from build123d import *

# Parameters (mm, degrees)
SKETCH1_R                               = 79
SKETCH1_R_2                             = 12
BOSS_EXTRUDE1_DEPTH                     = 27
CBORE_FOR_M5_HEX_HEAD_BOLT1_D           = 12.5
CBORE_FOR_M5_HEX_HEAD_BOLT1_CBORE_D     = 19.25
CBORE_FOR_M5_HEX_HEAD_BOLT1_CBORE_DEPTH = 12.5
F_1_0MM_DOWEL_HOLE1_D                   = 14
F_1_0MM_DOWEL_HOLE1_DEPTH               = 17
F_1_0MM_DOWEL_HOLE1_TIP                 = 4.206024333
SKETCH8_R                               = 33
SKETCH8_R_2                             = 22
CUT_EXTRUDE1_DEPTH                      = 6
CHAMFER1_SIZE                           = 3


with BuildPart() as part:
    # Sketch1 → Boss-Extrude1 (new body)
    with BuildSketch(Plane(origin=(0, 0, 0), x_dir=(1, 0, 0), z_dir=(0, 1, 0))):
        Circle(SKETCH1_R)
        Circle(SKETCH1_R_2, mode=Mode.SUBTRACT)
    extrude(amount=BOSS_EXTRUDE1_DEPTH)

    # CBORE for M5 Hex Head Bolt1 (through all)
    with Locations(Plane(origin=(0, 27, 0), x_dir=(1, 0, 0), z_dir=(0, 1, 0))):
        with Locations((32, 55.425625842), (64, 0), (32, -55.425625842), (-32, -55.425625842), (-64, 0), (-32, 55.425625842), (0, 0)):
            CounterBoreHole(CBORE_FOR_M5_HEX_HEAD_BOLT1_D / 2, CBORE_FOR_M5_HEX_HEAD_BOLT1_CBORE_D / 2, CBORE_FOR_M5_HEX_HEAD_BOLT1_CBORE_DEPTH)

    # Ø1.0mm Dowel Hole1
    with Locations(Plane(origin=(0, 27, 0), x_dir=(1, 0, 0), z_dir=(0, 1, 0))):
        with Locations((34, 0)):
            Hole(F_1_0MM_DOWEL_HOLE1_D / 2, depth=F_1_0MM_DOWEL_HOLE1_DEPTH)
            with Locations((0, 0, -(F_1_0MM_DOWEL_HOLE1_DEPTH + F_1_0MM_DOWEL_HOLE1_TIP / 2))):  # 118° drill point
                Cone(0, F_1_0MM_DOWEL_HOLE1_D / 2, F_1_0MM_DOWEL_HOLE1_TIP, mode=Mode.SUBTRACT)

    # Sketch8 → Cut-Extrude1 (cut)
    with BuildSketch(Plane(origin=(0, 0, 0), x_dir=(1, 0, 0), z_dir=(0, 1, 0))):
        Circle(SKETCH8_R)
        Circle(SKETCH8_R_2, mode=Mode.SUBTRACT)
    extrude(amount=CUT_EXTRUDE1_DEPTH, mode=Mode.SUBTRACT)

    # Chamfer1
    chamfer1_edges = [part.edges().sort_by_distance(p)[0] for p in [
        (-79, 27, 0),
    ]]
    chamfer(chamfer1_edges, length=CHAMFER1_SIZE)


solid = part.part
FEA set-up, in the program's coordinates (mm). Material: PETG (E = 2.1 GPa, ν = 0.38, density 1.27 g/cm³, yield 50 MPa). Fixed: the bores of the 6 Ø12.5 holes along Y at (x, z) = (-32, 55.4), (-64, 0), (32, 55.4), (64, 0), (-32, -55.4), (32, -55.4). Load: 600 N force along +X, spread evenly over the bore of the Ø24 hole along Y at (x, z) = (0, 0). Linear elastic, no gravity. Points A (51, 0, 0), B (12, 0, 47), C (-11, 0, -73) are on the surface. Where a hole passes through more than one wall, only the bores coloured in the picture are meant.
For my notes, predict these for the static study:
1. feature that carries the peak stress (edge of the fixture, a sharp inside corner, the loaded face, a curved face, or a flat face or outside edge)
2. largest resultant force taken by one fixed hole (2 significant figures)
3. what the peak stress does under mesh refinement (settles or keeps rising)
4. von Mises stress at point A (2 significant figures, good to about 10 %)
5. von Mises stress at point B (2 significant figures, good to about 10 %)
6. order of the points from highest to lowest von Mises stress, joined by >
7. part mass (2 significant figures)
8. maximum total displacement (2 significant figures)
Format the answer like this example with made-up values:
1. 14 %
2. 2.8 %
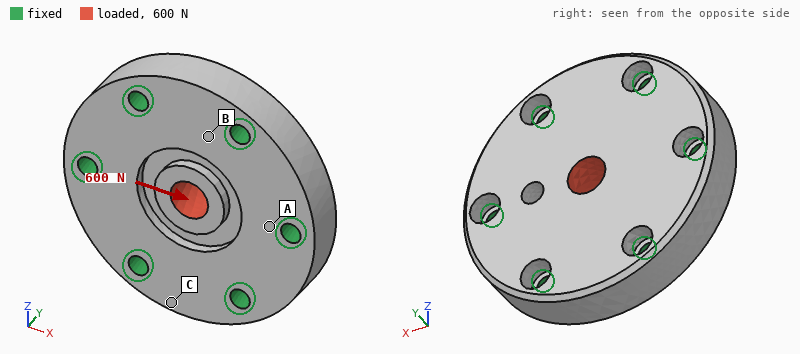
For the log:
1. a sharp inside corner
2. 150 N
3. keeps rising
4. 0.23 MPa
5. 0.12 MPa
6. A > B > C
7. 590 g
8. 10 µm
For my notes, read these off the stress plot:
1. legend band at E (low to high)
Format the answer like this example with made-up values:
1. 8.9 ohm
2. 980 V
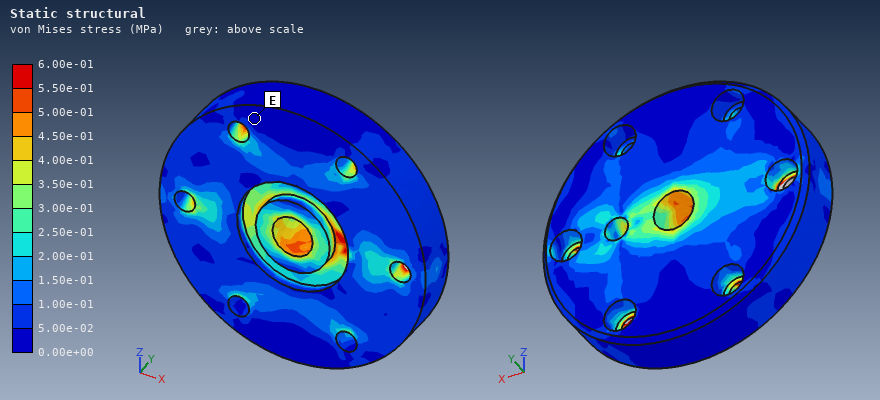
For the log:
1. 0.00e+00 to 5.00e-02 MPa
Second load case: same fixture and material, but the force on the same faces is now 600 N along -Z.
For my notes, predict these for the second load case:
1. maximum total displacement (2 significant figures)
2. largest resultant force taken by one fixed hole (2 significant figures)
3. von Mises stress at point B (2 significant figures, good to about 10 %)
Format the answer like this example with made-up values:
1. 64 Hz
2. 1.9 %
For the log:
1. 9.7 µm
2. 130 N
3. 0.100 MPa
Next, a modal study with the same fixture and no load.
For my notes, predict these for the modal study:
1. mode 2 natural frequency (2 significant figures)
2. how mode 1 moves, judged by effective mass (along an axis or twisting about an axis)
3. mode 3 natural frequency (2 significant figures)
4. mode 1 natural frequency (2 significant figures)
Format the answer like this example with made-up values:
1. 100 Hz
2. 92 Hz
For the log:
1. 3600 Hz
2. along Y
3. 3600 Hz
4. 2300 Hz
